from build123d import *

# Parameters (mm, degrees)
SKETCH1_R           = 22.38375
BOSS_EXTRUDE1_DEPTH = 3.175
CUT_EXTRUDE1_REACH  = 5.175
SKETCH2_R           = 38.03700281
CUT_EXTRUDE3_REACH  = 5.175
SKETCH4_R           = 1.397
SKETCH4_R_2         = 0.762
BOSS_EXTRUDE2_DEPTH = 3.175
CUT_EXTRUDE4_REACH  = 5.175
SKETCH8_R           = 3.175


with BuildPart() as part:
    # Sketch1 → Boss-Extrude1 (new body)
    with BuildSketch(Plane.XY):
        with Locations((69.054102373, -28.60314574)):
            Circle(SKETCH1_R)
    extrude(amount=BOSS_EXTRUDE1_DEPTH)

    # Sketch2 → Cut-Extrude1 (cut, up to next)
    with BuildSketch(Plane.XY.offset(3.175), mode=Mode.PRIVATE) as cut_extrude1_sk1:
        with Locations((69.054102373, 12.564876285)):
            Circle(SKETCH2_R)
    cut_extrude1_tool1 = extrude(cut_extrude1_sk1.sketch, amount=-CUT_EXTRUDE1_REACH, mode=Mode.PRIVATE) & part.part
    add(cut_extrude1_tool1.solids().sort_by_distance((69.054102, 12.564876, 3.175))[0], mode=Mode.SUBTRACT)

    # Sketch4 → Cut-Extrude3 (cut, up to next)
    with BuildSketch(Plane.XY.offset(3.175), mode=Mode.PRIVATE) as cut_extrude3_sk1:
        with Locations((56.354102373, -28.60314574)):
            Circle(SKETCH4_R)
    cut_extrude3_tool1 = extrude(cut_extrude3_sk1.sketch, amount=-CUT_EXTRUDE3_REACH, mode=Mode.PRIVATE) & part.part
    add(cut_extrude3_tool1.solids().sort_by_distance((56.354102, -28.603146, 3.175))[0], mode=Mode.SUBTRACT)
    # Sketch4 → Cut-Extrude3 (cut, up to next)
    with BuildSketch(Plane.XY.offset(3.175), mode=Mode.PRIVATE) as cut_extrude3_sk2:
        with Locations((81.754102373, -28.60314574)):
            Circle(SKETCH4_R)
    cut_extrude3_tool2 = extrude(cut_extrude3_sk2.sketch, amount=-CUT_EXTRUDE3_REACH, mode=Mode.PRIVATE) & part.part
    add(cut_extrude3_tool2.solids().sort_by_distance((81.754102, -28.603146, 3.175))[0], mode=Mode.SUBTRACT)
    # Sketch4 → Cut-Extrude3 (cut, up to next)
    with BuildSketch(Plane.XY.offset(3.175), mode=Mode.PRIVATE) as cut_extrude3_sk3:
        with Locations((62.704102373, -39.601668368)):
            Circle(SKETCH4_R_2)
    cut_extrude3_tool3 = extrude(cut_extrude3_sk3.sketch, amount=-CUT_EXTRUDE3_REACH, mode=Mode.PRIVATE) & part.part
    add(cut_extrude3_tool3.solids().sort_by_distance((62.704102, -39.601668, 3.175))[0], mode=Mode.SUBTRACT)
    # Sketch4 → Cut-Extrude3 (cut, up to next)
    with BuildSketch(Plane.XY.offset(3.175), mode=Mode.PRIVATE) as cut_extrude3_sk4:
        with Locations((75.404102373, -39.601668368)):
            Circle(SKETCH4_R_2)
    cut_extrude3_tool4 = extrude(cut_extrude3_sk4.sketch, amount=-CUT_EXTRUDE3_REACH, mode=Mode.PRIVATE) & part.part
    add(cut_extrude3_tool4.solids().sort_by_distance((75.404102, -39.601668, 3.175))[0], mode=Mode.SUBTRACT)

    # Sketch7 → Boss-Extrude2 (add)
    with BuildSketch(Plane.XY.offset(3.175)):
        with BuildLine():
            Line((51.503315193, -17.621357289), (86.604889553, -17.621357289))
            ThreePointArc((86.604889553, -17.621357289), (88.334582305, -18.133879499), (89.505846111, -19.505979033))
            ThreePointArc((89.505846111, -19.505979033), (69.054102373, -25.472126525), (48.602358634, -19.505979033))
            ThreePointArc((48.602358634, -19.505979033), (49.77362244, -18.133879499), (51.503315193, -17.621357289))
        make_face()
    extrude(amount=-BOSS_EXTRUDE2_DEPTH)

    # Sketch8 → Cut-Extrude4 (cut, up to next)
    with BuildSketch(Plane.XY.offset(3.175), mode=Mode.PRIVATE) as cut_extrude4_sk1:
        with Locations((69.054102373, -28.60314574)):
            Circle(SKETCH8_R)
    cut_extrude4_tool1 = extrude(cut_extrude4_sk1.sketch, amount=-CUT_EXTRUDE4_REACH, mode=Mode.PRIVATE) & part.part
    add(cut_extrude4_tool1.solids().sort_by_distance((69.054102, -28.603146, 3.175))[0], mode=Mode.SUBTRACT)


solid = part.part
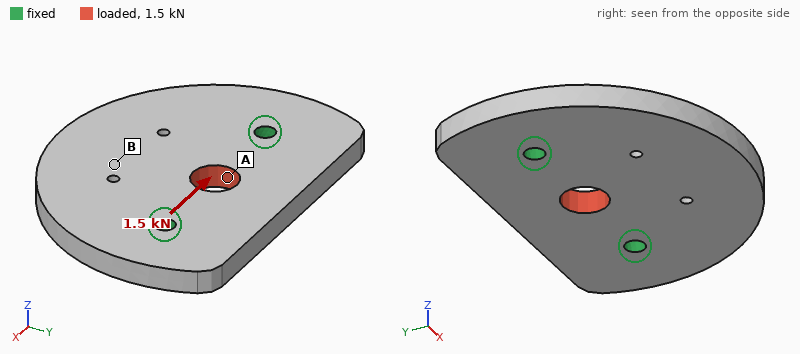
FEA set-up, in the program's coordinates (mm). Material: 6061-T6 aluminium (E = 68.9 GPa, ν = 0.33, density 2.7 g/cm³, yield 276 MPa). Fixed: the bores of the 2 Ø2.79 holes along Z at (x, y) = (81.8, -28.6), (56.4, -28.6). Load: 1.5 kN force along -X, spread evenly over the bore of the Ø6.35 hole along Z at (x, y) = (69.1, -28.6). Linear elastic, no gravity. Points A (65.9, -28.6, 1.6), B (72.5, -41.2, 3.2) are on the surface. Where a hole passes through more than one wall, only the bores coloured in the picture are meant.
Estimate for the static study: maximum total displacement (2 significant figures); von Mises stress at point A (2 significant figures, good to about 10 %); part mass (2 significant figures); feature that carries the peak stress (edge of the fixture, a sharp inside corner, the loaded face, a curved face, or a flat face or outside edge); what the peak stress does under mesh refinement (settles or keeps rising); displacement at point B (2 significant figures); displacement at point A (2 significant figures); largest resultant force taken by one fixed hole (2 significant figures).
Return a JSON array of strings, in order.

["4.1 µm", "24 MPa", "10 g", "edge of the fixture", "keeps rising", "1.8 µm", "3.4 µm", "750 N"]
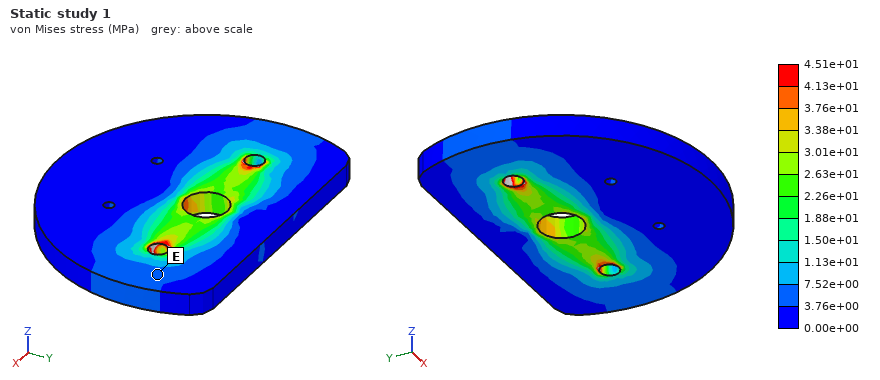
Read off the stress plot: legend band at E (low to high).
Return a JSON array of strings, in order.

["3.76e+00 to 7.52e+00 MPa"]
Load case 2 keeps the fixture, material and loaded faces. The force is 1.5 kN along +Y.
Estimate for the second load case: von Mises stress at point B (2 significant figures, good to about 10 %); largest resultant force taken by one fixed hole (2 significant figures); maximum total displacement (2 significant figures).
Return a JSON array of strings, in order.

["8.8 MPa", "750 N", "7.2 µm"]
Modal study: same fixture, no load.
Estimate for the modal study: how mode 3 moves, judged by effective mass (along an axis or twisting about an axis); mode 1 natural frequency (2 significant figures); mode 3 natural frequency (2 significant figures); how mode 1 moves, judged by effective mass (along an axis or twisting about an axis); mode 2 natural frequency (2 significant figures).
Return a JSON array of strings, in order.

["along Z", "5700 Hz", "16 kHz", "along Z", "12 kHz"]
